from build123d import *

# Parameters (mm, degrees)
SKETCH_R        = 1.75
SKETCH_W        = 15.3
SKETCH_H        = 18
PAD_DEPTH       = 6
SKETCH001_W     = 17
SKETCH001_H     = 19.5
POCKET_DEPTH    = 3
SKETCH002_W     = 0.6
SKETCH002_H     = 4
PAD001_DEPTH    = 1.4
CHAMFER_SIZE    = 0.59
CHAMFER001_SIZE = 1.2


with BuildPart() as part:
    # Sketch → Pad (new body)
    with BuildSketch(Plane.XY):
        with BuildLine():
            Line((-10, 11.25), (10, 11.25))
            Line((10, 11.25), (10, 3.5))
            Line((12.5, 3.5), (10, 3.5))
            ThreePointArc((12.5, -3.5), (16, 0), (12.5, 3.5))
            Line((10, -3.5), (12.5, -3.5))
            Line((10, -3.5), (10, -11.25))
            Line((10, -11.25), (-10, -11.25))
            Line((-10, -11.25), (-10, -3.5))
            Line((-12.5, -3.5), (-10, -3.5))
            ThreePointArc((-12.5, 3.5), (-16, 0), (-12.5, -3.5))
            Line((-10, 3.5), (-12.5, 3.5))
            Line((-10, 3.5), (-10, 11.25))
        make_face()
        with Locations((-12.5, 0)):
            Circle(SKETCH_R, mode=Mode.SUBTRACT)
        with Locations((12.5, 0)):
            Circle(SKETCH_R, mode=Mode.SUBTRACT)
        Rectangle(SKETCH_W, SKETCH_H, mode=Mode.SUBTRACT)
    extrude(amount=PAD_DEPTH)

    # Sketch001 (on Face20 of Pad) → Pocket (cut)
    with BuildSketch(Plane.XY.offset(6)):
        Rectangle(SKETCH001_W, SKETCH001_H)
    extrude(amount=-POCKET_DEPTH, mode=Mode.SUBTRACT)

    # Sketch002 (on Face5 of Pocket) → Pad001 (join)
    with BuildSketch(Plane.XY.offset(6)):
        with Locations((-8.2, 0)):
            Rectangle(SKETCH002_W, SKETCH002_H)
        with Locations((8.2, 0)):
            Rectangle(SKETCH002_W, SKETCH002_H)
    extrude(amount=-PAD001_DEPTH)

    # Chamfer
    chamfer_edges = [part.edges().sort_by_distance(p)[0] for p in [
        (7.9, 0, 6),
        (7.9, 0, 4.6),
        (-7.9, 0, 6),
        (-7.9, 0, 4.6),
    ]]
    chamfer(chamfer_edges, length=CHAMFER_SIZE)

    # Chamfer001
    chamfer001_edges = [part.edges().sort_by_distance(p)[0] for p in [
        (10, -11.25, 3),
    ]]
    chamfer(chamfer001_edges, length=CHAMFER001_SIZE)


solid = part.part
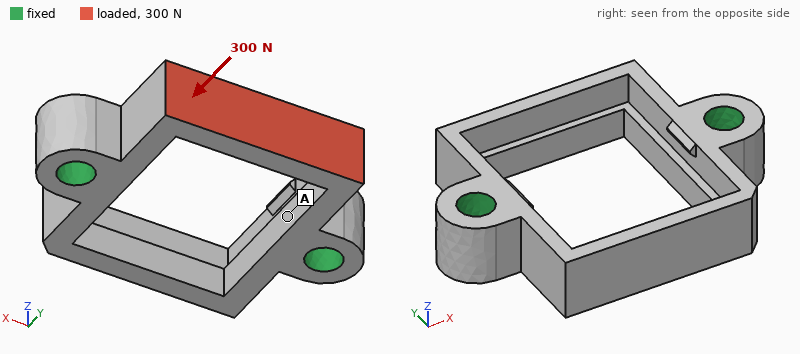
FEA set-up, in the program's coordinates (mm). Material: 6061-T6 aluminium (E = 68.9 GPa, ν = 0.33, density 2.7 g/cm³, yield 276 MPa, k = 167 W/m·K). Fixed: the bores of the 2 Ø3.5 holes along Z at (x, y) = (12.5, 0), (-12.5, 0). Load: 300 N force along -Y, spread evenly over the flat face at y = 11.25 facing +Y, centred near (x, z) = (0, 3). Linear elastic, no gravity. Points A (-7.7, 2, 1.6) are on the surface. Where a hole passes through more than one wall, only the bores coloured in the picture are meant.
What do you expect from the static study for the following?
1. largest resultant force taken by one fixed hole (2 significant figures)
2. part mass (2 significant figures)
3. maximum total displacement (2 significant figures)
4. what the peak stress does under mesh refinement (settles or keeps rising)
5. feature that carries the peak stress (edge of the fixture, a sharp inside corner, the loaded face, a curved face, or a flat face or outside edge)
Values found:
170 N
3.3 g
34 µm
keeps rising
a sharp inside corner
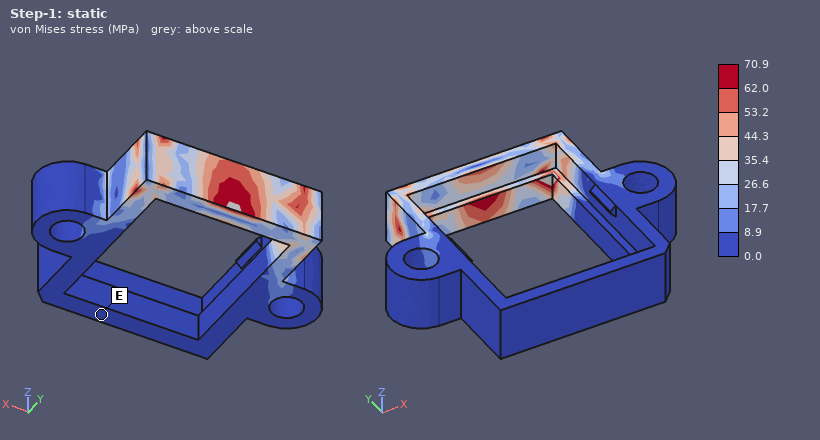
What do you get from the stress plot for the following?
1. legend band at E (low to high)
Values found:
0.0 to 8.9 MPa
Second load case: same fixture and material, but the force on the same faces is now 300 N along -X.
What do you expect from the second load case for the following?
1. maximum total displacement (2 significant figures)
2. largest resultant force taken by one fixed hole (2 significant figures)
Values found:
45 µm
170 N
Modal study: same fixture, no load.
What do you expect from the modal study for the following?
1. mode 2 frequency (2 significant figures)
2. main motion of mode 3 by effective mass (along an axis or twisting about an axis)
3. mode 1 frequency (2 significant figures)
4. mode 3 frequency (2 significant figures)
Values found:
17 kHz
twisting about X
16 kHz
19 kHz
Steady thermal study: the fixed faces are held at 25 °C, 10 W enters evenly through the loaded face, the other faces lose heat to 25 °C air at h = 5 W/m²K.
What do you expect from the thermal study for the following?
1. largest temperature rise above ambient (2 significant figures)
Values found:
32 K
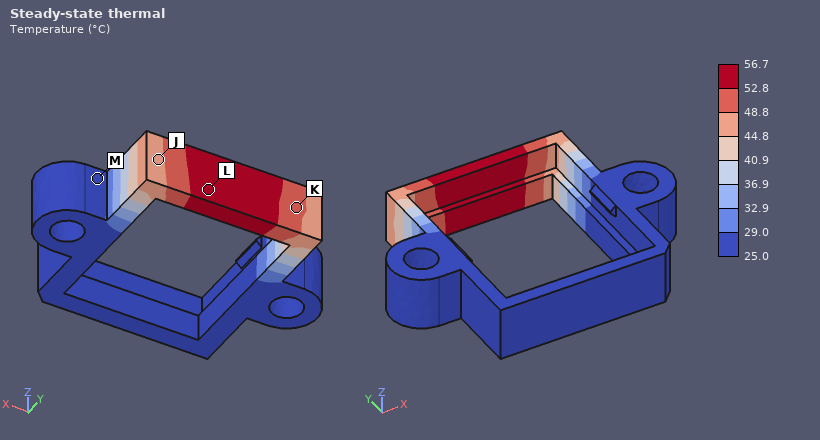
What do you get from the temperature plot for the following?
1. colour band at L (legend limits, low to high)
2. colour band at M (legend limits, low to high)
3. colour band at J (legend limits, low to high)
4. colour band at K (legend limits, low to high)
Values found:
52.8 to 56.7 °C
25.0 to 29.0 °C
44.8 to 48.8 °C
48.8 to 52.8 °C
